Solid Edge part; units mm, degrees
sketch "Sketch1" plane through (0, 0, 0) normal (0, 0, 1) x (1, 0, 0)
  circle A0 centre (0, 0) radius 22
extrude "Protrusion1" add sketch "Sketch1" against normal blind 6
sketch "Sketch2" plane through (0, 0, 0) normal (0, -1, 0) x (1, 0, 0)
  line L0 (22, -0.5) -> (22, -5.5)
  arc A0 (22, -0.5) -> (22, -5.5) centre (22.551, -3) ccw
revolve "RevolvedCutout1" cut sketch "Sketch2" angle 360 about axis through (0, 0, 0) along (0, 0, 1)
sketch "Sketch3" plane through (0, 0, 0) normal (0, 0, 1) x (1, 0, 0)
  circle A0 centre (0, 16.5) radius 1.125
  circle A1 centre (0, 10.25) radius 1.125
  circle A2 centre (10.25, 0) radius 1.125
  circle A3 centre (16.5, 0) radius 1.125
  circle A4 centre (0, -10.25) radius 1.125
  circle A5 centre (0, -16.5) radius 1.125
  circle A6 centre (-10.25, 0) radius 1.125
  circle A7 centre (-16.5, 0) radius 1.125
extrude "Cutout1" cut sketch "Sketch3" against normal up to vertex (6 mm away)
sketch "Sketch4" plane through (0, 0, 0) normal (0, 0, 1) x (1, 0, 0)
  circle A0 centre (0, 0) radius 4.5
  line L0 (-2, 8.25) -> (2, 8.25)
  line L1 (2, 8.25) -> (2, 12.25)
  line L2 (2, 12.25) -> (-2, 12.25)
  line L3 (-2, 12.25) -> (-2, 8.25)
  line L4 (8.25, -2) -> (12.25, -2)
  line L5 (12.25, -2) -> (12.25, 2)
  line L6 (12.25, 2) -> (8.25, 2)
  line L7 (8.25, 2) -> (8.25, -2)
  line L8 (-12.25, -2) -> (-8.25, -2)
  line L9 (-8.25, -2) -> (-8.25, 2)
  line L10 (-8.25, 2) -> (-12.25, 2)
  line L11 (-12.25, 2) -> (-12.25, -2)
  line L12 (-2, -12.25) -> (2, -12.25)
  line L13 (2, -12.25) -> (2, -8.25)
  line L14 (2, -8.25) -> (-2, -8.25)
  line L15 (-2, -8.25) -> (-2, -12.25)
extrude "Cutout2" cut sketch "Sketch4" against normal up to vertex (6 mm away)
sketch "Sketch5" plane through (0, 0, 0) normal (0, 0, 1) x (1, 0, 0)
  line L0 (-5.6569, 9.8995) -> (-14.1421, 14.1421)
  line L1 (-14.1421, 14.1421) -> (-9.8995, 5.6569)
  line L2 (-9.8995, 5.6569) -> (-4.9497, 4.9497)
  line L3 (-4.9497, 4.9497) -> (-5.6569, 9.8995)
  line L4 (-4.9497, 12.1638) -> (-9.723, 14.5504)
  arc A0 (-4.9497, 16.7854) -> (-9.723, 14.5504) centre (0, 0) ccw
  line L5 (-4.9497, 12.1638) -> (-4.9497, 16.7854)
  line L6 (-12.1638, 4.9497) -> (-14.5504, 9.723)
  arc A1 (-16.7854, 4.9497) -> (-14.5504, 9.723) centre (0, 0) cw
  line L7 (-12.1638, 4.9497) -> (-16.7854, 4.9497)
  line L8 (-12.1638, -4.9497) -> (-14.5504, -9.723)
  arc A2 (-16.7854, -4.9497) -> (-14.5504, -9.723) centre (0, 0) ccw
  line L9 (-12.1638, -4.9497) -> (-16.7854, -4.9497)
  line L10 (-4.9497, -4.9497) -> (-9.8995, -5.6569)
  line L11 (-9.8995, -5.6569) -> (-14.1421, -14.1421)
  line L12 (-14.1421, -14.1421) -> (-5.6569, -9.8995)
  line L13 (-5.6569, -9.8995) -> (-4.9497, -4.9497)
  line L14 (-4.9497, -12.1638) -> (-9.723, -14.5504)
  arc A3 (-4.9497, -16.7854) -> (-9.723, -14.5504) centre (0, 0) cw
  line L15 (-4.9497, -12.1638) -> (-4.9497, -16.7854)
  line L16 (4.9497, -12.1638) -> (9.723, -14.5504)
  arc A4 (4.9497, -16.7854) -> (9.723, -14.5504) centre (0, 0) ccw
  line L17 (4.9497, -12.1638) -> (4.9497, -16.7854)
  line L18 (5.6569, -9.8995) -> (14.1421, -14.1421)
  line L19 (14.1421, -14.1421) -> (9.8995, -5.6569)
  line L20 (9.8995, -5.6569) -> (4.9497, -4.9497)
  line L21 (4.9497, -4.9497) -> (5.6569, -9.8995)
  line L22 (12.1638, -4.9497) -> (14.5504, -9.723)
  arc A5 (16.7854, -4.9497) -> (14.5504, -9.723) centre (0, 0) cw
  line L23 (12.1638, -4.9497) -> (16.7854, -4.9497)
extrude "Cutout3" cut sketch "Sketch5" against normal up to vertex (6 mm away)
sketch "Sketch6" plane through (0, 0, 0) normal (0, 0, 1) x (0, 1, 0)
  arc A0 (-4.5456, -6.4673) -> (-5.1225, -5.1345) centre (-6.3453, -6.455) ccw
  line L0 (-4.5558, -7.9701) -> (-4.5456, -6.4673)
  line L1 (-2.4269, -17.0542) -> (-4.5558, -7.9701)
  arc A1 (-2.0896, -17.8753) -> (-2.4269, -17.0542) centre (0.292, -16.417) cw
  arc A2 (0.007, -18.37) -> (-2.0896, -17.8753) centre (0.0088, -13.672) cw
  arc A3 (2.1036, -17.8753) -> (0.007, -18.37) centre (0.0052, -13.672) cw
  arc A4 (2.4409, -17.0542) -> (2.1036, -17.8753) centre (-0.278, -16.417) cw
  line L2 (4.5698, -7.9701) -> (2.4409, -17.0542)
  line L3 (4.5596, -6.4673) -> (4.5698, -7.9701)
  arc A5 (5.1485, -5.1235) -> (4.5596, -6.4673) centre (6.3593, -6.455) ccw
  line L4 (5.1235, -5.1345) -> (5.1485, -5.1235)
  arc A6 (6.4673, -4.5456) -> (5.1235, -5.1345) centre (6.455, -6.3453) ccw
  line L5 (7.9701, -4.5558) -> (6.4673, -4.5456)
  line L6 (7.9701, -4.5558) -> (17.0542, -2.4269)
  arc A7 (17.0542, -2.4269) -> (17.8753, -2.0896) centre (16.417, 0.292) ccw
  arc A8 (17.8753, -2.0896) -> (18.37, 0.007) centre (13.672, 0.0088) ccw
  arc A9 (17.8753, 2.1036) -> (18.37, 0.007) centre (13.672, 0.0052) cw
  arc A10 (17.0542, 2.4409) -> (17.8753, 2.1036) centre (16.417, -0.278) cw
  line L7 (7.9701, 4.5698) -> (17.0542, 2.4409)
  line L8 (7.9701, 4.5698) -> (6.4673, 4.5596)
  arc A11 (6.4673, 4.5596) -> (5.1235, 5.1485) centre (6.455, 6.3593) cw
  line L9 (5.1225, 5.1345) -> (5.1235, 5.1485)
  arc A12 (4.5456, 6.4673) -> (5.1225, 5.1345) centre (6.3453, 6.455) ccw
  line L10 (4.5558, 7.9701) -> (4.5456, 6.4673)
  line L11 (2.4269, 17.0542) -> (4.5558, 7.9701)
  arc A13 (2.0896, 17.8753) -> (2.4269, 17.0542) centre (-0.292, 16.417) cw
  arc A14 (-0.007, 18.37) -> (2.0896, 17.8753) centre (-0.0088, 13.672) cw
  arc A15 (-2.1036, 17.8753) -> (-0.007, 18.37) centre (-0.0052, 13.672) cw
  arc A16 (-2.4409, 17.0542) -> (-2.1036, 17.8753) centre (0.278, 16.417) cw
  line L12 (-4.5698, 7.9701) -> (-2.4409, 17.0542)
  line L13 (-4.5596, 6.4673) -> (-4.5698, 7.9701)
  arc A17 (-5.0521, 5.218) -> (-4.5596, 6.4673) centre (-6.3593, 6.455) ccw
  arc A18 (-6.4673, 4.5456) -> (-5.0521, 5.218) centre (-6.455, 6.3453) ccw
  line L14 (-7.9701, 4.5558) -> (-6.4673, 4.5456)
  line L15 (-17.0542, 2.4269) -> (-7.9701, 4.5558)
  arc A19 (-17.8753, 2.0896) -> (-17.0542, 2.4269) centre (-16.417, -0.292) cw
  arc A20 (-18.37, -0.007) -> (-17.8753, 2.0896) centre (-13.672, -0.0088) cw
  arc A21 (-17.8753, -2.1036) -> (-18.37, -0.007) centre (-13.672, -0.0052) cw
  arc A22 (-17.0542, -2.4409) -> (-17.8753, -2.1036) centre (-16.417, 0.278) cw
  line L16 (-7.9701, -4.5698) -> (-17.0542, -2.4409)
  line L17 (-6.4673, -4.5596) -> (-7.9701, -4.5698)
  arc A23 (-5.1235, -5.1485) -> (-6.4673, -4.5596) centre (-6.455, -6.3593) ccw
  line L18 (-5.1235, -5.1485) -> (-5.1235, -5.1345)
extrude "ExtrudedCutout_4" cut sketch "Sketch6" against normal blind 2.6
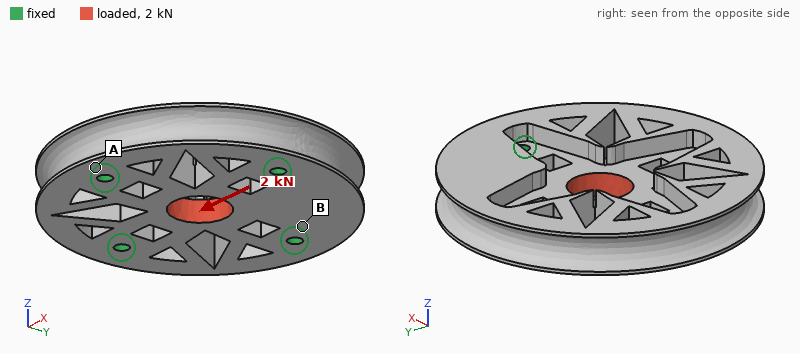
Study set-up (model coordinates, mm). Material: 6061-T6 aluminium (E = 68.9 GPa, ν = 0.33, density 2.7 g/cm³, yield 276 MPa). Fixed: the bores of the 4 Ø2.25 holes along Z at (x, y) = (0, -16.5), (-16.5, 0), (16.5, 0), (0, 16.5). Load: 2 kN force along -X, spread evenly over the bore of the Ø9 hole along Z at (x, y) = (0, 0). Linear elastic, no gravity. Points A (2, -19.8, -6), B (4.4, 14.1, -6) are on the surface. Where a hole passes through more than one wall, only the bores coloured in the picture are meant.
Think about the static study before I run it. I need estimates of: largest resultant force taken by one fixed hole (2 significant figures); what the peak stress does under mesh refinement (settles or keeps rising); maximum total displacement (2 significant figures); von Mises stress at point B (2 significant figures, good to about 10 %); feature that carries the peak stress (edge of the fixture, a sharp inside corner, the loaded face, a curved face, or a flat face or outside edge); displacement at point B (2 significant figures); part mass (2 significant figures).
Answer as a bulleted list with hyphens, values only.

- 660 N
- keeps rising
- 7.1 µm
- 11 MPa
- a sharp inside corner
- 1.1 µm
- 14 g
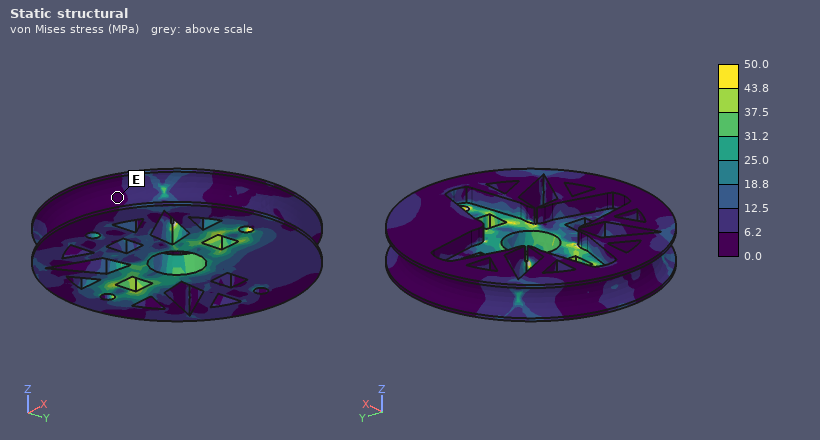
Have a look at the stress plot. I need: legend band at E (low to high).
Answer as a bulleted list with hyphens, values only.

- 0.0 to 6.2 MPa
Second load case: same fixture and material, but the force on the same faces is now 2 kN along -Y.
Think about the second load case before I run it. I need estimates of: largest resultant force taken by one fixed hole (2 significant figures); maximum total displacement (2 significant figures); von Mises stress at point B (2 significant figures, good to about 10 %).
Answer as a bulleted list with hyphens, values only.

- 660 N
- 7.1 µm
- 18 MPa
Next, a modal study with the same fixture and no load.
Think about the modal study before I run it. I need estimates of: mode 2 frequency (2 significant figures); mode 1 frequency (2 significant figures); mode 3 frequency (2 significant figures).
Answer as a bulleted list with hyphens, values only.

- 20 kHz
- 17 kHz
- 21 kHz
